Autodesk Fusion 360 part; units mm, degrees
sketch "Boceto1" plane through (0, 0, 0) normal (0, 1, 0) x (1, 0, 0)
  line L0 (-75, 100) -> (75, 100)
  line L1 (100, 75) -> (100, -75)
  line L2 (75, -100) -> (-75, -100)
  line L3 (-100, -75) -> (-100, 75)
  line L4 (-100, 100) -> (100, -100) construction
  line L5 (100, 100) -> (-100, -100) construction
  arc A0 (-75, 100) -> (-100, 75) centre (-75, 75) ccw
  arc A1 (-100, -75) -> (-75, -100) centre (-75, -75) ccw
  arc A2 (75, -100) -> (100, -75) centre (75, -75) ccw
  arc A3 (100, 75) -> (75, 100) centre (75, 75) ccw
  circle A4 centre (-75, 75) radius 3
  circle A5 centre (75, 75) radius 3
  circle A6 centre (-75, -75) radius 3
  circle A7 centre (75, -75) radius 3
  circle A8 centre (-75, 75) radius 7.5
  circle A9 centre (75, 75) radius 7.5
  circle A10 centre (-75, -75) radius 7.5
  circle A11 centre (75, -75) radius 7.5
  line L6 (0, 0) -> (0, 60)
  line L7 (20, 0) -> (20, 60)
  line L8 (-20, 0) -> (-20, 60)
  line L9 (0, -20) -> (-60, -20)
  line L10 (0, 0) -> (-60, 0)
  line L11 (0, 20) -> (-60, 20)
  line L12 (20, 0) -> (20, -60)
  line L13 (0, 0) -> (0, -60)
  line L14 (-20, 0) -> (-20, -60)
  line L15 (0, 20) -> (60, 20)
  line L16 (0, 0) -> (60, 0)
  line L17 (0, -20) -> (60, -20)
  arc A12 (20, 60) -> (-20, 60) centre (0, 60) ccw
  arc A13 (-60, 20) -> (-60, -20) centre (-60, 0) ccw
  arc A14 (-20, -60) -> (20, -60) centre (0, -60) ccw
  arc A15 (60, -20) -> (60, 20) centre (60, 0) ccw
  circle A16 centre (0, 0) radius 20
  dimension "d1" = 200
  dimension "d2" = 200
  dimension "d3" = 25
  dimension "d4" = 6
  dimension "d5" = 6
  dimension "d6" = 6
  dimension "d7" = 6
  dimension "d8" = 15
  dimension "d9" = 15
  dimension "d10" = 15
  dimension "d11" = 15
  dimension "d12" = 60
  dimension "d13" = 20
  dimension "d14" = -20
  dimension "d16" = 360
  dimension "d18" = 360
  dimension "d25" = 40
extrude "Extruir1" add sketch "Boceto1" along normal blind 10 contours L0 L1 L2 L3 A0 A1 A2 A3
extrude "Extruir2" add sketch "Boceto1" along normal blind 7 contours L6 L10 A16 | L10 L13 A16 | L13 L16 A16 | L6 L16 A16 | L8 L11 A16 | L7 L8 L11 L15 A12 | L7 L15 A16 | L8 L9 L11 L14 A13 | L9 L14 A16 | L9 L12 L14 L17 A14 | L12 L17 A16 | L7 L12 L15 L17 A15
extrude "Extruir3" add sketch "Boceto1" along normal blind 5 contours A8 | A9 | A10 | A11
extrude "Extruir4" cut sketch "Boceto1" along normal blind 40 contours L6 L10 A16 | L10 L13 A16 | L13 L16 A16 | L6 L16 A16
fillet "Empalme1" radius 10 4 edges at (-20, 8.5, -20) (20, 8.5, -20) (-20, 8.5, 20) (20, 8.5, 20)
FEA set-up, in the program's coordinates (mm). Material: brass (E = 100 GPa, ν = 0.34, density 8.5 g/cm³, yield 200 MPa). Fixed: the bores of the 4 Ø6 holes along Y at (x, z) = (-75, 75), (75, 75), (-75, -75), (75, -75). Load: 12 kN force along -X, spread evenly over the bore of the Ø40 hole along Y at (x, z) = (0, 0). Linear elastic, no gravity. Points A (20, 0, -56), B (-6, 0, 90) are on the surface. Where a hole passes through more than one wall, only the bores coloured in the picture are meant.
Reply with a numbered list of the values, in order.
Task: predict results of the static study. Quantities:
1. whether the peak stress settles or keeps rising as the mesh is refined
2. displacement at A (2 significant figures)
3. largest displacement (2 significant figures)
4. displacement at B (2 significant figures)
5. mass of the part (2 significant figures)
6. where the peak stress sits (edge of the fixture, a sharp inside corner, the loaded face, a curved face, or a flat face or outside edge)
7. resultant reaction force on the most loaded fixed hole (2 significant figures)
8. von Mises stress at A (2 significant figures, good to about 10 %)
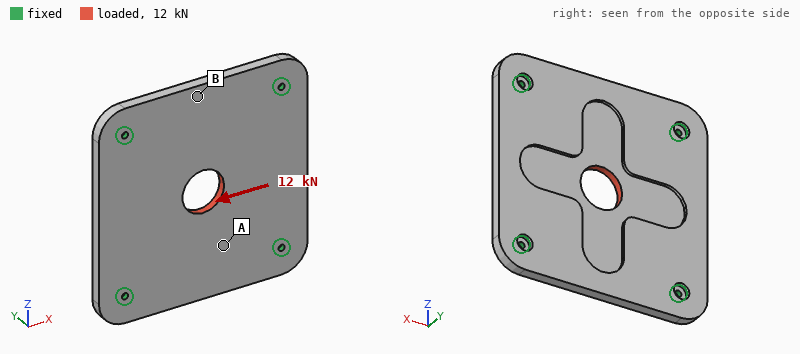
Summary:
1. keeps rising
2. 6.5 µm
3. 13 µm
4. 4.3 µm
5. 3.0 kg
6. edge of the fixture
7. 3.2 kN
8. 6.4 MPa
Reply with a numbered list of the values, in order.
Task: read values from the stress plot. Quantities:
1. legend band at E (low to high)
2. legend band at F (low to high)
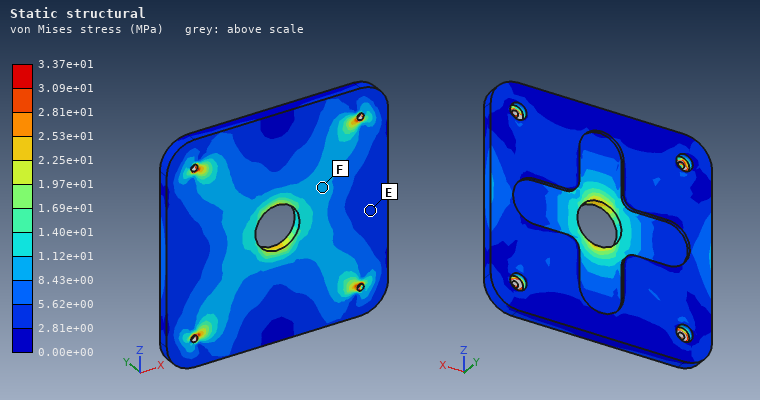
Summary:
1. 2.81e+00 to 5.62e+00 MPa
2. 8.43e+00 to 1.12e+01 MPa
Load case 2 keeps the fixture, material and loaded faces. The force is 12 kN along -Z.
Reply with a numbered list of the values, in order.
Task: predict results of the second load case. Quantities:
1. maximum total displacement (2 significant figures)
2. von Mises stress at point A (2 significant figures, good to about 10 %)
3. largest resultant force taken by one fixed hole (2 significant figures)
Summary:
1. 13 µm
2. 7.5 MPa
3. 3.2 kN
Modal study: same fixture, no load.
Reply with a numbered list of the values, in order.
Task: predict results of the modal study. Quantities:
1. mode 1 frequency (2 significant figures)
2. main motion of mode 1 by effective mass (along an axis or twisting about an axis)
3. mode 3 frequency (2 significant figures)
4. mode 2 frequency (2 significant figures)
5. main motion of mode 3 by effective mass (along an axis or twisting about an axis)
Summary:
1. 730 Hz
2. along Y
3. 1200 Hz
4. 1000 Hz
5. twisting about X
